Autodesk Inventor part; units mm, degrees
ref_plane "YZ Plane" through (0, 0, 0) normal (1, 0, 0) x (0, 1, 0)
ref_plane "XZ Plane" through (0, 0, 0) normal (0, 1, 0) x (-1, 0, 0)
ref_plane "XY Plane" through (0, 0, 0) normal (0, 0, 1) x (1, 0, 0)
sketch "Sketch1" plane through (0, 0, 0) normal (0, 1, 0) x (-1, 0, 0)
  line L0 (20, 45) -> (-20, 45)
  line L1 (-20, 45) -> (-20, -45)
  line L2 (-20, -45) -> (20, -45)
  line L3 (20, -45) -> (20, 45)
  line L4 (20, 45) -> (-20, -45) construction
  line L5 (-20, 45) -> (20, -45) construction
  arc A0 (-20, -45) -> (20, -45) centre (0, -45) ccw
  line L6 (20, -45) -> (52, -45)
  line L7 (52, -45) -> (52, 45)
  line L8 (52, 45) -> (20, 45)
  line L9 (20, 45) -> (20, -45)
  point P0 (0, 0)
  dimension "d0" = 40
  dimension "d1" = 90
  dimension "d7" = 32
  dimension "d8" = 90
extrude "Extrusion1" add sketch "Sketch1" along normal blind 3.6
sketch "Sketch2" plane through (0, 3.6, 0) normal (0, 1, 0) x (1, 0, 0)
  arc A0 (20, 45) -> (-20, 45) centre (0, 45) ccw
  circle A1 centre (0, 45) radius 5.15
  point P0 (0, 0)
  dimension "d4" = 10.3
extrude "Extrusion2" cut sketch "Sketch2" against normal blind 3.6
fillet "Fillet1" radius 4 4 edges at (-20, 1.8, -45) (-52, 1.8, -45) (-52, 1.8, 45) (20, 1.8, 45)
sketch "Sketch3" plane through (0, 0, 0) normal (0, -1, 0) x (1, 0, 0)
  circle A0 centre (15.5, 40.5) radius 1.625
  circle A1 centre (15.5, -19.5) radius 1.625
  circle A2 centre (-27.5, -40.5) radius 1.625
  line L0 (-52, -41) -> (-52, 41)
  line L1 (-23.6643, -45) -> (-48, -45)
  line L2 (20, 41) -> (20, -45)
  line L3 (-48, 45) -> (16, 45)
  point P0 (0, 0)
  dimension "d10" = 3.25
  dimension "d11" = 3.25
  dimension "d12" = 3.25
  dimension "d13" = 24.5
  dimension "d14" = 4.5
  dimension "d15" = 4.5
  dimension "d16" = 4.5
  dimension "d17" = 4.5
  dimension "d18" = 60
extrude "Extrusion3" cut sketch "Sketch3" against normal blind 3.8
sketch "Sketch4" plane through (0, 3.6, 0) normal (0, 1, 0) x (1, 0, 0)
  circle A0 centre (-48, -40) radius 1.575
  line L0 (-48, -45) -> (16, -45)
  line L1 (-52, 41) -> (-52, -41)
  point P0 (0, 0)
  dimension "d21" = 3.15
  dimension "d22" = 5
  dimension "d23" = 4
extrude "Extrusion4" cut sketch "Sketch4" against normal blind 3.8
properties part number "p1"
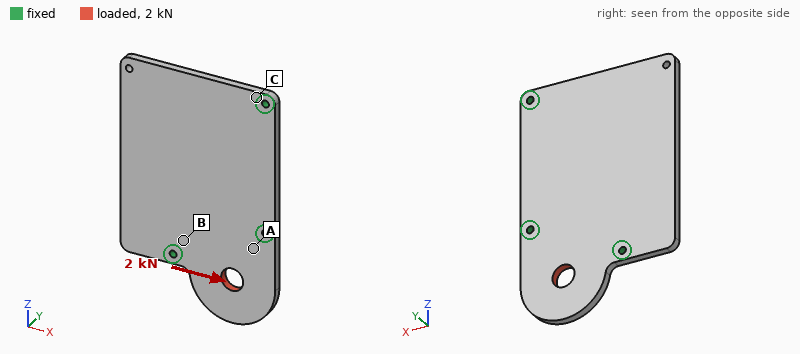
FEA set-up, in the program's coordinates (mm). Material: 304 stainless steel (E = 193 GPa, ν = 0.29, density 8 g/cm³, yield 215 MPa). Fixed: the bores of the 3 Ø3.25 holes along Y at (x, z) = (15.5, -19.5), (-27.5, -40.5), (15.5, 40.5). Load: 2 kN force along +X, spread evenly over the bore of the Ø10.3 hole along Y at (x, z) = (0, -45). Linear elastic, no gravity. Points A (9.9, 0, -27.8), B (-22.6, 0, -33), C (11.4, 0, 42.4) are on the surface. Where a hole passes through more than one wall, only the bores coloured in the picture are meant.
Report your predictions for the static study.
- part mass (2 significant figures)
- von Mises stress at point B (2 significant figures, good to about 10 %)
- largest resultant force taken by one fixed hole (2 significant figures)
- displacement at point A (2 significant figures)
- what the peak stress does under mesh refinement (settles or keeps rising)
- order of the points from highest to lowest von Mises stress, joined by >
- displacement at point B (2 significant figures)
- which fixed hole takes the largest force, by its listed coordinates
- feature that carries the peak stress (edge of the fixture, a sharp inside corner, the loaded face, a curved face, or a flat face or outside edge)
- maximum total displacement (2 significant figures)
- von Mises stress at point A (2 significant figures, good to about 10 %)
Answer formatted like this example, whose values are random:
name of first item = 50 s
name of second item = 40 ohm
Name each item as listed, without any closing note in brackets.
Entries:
part mass = 200 g
von Mises stress at point B = 8.4 MPa
largest resultant force taken by one fixed hole = 1.4 kN
displacement at point A = 1.3 µm
what the peak stress does under mesh refinement = keeps rising
order of the points from highest to lowest von Mises stress, joined by > = A > B > C
displacement at point B = 1.2 µm
which fixed hole takes the largest force, by its listed coordinates = (-27.5, -40.5)
feature that carries the peak stress = edge of the fixture
maximum total displacement = 5.8 µm
von Mises stress at point A = 14 MPa
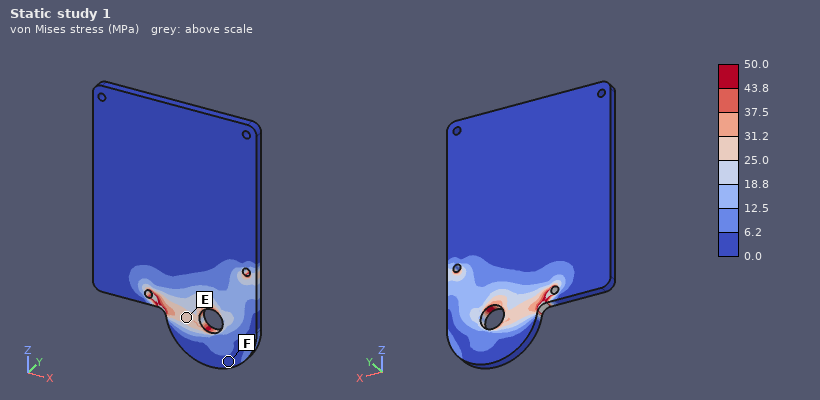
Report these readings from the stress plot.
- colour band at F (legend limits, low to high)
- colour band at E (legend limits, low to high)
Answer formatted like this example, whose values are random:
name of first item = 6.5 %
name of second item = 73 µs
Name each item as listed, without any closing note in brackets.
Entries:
colour band at F = 0.0 to 6.2 MPa
colour band at E = 25.0 to 31.2 MPa
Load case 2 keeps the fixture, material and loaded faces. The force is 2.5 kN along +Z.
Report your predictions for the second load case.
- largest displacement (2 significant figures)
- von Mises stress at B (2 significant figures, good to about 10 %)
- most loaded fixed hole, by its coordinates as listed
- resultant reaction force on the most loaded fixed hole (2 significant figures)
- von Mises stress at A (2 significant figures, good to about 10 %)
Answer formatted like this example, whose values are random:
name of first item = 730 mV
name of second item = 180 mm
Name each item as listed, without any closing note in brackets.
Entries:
largest displacement = 4.8 µm
von Mises stress at B = 13 MPa
most loaded fixed hole, by its coordinates as listed = (15.5, -19.5)
resultant reaction force on the most loaded fixed hole = 1.5 kN
von Mises stress at A = 23 MPa
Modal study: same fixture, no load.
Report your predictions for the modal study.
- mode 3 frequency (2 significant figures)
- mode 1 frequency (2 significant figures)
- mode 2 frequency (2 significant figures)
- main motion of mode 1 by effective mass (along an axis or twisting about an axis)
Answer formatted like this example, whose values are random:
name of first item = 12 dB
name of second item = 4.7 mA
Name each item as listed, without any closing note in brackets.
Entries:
mode 3 frequency = 2700 Hz
mode 1 frequency = 850 Hz
mode 2 frequency = 2100 Hz
main motion of mode 1 by effective mass = along Y
